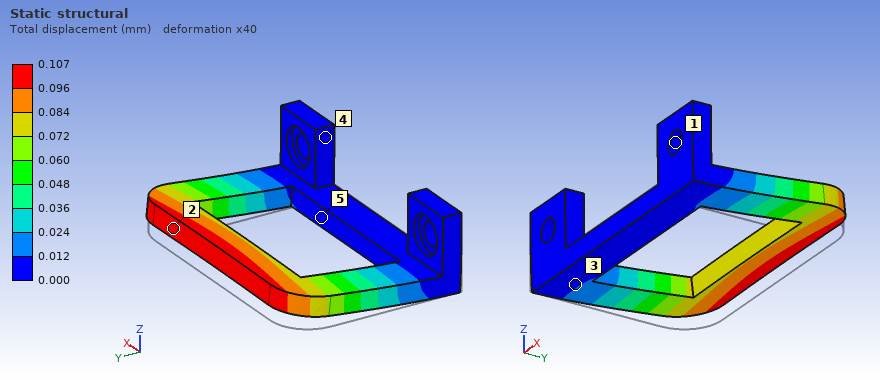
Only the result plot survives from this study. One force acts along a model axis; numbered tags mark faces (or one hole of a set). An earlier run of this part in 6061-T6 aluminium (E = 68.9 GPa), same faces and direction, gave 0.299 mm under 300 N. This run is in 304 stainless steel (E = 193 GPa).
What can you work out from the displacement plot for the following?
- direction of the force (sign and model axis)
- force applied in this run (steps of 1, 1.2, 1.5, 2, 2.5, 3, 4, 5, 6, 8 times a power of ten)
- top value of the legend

+Z
300 N
0.107 mm
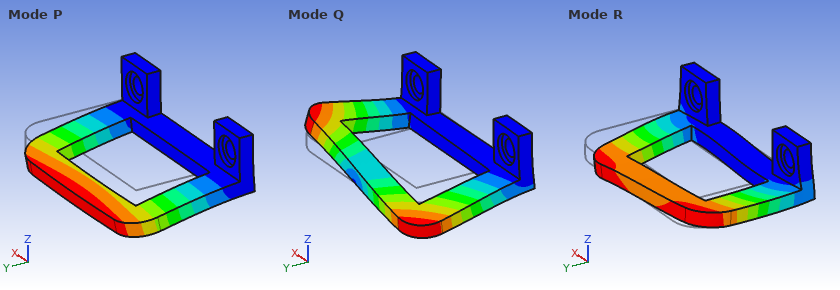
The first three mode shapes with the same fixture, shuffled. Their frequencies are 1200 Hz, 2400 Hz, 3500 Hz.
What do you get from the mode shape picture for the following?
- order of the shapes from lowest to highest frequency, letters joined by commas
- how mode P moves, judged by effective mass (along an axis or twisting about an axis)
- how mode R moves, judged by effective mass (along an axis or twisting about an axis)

P, Q, R
along Z
along X
